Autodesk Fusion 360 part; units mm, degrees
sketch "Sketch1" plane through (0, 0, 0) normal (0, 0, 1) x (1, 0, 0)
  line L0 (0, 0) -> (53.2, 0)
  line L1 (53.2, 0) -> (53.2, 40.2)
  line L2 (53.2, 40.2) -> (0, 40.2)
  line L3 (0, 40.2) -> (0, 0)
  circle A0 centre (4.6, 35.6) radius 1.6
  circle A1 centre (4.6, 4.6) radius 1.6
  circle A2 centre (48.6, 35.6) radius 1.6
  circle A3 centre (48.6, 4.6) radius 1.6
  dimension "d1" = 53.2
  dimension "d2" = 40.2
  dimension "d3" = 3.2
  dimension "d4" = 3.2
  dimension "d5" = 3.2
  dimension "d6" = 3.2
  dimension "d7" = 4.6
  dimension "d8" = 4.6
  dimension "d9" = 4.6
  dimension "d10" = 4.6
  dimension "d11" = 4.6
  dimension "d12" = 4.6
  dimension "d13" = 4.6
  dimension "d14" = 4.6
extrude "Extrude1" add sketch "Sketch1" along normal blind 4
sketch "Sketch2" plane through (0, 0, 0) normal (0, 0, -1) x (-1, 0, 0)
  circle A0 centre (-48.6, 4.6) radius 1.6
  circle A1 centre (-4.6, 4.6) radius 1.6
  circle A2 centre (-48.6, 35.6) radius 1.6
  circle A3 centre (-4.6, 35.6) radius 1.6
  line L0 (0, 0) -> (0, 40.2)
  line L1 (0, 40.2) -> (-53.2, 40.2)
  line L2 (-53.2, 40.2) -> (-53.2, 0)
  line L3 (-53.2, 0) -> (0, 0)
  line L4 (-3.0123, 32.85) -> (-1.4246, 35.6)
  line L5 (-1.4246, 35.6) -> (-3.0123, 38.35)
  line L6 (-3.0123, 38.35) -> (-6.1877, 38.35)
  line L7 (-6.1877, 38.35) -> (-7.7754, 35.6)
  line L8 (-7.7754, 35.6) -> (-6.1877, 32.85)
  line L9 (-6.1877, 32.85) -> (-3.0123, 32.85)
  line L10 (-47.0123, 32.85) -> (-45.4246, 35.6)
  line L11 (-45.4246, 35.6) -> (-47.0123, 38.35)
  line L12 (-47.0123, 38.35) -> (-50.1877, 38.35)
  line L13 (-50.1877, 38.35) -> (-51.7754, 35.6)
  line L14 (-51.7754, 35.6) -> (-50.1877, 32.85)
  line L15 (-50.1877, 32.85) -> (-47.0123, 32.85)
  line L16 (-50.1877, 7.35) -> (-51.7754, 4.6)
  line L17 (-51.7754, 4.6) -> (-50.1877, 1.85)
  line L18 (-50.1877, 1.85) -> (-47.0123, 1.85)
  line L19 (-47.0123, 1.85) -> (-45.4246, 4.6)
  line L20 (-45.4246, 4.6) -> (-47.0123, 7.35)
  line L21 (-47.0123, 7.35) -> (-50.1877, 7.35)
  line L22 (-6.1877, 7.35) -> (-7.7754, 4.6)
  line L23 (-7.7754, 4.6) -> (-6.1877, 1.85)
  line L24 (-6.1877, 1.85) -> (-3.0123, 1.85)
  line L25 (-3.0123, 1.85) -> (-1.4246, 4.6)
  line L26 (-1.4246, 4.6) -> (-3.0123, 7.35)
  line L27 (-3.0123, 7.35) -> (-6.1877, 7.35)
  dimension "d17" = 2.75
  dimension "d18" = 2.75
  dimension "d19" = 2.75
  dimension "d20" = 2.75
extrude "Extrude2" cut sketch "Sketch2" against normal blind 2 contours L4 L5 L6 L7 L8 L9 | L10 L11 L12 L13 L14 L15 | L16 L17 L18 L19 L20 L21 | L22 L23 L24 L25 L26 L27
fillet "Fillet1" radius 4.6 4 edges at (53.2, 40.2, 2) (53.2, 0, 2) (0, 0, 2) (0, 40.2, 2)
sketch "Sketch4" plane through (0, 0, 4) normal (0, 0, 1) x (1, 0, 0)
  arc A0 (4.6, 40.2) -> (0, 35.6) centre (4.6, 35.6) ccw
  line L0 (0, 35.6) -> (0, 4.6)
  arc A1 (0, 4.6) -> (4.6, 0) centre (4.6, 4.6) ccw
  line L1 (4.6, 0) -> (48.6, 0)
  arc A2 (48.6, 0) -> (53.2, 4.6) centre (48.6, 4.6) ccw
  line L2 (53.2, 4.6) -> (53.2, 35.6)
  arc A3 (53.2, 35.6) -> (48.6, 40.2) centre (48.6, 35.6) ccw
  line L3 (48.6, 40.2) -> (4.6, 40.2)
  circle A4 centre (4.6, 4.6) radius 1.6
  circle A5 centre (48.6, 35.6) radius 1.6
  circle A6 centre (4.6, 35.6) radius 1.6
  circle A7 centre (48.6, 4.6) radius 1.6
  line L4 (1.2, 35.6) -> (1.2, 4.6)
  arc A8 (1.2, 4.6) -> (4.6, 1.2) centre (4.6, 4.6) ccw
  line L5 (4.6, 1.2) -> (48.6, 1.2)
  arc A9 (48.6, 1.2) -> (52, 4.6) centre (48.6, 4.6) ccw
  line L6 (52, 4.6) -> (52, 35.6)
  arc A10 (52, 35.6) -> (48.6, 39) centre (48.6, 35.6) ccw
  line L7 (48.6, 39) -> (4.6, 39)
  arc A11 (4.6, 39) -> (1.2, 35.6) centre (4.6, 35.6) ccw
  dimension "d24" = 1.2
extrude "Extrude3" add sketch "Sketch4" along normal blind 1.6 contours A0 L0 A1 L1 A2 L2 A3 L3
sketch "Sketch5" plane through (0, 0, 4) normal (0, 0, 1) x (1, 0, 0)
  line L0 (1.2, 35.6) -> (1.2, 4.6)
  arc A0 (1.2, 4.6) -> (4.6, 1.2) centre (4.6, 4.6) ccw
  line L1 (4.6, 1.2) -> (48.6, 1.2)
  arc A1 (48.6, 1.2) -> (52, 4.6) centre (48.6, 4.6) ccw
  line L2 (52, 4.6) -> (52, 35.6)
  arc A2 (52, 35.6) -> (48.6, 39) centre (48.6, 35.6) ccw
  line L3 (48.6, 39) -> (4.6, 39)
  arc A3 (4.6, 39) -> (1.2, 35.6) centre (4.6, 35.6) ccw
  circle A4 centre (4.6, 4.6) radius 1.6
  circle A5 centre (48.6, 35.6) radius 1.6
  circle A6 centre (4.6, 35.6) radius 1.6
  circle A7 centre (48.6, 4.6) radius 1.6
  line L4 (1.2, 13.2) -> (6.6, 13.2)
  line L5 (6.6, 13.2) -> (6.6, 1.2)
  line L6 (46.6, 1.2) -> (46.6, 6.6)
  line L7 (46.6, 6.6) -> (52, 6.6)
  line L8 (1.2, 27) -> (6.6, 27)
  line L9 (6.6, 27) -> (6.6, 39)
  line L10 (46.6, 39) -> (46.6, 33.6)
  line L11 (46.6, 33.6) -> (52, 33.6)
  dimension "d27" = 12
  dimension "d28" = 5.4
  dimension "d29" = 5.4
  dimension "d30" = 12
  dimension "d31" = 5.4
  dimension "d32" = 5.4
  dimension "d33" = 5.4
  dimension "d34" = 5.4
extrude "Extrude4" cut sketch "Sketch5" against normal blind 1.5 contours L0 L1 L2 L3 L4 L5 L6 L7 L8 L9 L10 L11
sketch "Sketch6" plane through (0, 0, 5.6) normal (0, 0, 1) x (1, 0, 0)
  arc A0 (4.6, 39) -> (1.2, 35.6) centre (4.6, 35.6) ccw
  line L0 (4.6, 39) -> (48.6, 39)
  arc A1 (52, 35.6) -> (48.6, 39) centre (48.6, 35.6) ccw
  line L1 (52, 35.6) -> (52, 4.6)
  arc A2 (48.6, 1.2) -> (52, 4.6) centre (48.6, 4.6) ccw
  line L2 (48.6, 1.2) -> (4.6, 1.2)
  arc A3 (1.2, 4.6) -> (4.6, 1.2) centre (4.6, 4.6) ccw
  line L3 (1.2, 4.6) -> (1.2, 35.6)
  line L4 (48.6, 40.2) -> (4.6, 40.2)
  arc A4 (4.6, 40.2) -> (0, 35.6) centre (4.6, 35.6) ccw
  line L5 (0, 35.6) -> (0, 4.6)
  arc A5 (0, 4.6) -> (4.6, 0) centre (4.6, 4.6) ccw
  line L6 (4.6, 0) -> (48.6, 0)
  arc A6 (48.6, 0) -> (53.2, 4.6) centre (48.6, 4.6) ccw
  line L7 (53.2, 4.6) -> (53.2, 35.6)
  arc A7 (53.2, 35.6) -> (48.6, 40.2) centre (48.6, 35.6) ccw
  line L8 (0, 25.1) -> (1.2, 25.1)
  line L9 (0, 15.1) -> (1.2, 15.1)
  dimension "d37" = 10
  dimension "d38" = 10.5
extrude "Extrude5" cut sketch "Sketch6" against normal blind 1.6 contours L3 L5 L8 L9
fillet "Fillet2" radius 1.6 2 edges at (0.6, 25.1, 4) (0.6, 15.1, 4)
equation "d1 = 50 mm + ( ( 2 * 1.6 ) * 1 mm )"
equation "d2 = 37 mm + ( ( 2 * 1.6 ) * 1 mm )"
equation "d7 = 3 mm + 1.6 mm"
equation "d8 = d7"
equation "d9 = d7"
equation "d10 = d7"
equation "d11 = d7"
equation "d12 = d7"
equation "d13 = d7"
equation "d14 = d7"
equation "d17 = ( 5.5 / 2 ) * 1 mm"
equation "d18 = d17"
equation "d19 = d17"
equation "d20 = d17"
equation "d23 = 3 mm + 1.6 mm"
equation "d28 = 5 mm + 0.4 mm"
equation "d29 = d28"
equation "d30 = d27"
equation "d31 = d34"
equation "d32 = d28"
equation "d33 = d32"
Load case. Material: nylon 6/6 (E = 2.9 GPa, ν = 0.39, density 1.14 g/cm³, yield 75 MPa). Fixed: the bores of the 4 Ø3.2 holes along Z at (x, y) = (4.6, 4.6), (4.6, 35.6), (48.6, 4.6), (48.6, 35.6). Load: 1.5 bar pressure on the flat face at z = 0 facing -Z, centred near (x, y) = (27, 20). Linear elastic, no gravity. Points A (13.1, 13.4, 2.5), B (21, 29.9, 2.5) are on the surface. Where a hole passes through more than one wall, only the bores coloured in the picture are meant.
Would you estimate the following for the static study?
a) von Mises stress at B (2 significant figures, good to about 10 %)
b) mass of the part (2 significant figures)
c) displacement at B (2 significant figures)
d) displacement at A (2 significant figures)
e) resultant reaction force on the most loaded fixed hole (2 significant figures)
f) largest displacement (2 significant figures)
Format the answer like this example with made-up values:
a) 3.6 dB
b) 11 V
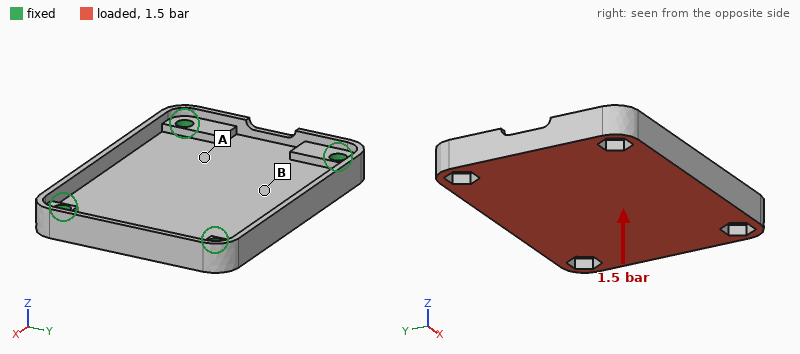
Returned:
a) 6.7 MPa
b) 6.8 g
c) 0.39 mm
d) 0.26 mm
e) 140 N
f) 0.49 mm
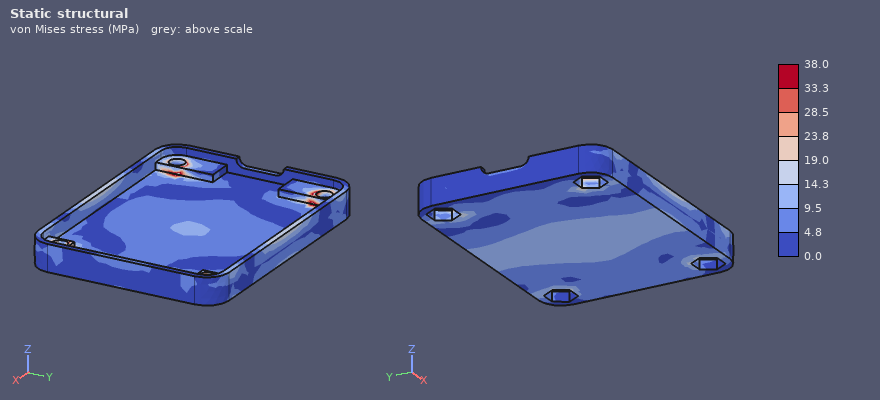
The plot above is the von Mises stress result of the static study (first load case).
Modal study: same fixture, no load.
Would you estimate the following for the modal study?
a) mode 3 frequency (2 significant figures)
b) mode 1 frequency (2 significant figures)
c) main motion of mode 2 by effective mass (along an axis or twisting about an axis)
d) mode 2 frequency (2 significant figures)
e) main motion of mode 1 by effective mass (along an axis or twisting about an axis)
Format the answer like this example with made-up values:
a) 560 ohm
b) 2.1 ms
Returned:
a) 3800 Hz
b) 1900 Hz
c) twisting about X
d) 2800 Hz
e) along Z
